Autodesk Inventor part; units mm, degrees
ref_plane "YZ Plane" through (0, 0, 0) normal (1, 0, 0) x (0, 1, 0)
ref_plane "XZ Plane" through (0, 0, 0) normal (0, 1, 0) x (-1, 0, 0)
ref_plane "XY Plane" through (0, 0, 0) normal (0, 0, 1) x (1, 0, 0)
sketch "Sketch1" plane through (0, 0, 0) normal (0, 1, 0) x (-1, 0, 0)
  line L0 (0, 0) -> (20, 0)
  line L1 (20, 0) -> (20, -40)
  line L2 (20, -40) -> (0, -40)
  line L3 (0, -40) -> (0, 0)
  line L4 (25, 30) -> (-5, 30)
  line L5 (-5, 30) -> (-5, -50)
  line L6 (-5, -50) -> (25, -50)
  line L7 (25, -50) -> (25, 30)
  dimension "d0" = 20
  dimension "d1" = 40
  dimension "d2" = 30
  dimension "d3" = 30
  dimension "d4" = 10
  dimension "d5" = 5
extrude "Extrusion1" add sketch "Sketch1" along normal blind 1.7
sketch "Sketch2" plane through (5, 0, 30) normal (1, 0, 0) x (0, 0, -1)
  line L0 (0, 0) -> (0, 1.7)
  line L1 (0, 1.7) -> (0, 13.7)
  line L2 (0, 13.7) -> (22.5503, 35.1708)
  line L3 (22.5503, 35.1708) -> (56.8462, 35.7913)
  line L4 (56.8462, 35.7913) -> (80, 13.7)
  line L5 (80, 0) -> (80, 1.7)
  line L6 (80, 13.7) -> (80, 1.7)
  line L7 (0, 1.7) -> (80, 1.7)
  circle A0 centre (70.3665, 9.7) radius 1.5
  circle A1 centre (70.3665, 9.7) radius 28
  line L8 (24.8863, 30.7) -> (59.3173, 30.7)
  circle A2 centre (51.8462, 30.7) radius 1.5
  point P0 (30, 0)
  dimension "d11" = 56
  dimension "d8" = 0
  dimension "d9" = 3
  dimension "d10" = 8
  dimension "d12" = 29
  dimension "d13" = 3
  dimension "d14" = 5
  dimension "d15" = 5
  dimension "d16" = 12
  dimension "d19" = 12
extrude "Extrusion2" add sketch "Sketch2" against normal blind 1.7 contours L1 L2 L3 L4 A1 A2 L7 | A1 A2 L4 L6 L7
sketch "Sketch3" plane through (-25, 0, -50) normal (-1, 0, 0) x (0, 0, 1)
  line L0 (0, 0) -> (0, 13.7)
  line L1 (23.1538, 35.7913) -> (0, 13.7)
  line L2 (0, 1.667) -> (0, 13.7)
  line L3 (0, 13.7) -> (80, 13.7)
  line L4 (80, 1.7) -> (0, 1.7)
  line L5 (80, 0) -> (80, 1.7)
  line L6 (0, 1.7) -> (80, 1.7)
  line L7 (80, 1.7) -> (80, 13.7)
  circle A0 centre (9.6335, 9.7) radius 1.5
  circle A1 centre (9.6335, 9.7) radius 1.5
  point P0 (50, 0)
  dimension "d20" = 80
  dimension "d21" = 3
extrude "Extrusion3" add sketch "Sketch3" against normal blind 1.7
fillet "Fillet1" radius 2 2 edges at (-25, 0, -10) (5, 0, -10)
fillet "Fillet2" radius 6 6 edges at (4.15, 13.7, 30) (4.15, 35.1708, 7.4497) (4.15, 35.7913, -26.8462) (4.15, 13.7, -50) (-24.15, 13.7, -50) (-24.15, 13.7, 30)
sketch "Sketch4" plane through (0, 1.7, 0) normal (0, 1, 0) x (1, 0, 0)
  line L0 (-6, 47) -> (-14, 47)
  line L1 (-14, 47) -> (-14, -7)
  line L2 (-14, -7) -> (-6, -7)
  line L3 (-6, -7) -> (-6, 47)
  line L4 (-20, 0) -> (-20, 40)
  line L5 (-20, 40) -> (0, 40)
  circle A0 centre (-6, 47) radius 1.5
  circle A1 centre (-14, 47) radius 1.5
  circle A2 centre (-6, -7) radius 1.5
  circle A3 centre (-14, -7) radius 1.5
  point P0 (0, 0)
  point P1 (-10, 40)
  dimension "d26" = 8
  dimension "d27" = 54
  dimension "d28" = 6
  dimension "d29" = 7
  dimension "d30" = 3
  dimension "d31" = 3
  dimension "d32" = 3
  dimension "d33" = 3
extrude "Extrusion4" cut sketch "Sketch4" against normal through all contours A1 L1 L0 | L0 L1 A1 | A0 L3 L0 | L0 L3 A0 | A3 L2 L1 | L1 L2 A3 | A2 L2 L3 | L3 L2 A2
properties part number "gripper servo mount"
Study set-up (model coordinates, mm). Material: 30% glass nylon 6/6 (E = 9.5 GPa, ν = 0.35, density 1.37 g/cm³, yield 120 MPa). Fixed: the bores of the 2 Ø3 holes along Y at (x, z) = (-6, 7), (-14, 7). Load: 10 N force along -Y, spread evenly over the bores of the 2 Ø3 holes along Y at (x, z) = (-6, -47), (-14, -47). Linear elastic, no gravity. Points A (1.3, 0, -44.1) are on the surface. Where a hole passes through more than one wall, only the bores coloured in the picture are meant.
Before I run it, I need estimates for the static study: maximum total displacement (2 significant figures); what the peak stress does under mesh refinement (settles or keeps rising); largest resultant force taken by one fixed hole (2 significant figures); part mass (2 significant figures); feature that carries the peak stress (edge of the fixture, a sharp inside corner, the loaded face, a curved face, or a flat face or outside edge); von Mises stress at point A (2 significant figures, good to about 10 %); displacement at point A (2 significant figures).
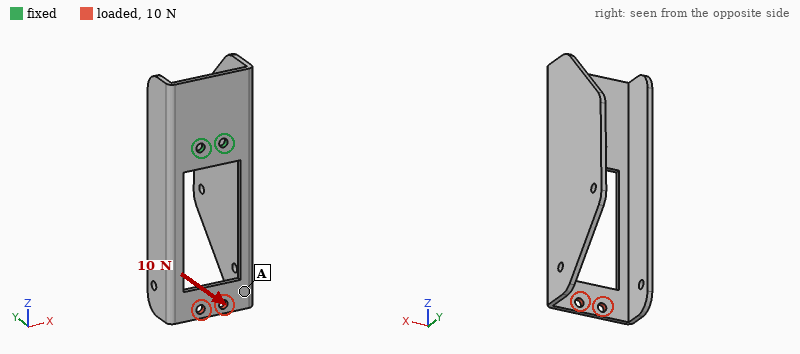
1.1 mm
keeps rising
5.8 N
11 g
edge of the fixture
3.7 MPa
0.91 mm
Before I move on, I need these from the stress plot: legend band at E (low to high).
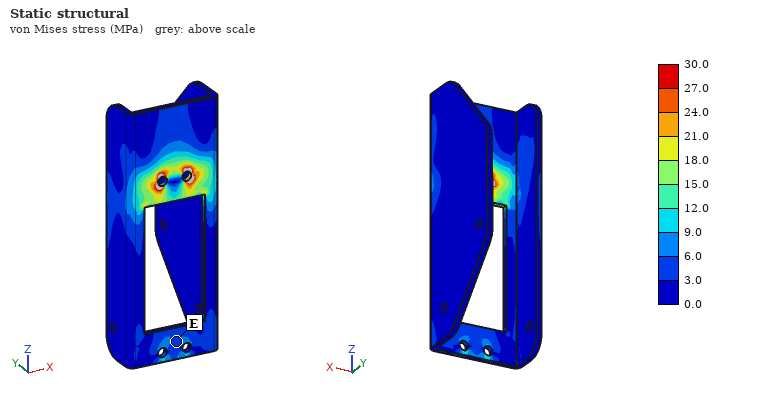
3.0 to 6.0 MPa
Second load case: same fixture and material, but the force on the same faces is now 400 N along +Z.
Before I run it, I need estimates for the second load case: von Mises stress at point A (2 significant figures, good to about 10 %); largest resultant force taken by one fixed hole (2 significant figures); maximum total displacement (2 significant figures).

23 MPa
200 N
0.32 mm
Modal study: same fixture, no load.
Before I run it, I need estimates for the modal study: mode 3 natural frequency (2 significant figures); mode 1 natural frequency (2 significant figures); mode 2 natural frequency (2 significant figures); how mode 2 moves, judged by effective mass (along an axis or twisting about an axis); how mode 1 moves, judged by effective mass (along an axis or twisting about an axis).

570 Hz
260 Hz
330 Hz
along X
along Y
